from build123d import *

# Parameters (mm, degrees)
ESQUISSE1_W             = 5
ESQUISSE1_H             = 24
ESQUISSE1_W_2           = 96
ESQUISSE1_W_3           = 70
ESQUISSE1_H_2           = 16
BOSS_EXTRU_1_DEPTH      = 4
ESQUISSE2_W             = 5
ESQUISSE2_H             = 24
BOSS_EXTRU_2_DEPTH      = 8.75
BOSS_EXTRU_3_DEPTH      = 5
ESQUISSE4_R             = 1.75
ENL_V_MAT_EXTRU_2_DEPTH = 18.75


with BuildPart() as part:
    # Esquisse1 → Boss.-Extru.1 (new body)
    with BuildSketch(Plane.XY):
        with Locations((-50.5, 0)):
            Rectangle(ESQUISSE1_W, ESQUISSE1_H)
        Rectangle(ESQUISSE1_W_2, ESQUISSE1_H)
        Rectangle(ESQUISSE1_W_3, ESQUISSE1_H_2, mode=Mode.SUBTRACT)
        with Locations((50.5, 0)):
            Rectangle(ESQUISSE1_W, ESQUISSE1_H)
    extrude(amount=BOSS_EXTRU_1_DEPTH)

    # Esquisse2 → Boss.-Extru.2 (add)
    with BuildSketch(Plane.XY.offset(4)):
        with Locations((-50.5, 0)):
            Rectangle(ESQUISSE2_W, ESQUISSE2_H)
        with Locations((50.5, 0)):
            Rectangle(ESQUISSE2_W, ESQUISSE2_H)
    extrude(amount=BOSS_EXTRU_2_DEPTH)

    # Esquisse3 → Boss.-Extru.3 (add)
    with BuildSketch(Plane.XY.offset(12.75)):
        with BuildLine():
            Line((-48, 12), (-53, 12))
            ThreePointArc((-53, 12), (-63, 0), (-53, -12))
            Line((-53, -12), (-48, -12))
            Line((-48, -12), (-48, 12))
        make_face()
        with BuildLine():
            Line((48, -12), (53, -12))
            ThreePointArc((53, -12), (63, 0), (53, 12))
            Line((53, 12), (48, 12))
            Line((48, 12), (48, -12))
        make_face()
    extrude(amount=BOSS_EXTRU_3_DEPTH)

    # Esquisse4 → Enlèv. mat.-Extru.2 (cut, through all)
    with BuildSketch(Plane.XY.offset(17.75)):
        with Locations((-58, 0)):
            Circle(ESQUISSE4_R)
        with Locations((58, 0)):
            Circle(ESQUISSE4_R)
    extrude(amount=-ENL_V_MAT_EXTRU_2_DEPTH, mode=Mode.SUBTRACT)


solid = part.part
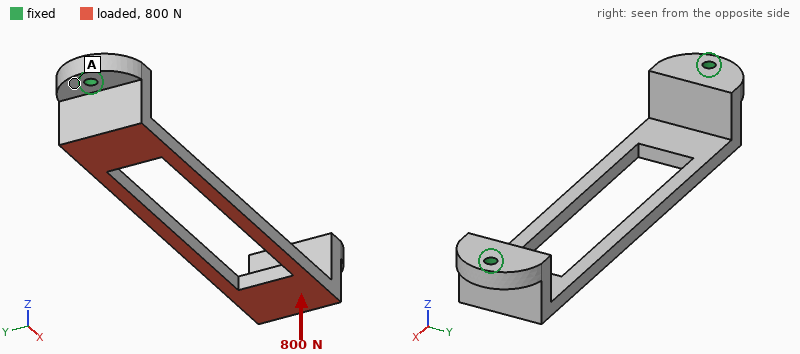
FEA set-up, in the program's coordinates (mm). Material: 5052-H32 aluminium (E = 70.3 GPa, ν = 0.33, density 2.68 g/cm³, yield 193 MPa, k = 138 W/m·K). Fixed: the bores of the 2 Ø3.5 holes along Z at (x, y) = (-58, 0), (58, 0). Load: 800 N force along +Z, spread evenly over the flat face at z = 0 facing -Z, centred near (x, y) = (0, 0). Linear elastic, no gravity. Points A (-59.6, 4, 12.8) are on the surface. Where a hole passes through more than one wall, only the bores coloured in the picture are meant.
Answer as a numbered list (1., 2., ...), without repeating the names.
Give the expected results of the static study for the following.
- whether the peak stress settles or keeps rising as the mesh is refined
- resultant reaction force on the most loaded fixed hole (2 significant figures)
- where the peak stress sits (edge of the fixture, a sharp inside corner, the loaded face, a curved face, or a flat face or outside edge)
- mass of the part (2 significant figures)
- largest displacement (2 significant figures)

1. keeps rising
2. 630 N
3. edge of the fixture
4. 29 g
5. 0.29 mm
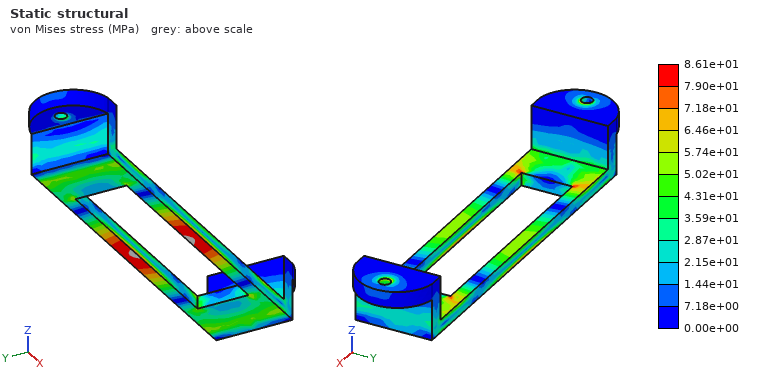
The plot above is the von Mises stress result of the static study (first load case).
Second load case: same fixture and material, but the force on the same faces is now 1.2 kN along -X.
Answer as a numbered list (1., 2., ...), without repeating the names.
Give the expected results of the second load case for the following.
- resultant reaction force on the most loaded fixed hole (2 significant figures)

1. 600 N
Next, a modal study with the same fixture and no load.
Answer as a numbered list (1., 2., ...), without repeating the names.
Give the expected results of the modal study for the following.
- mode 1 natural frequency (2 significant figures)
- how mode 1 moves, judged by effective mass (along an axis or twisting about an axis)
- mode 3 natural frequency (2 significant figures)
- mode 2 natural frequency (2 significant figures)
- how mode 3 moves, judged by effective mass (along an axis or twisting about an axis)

1. 2500 Hz
2. along Z
3. 3300 Hz
4. 2900 Hz
5. along Y
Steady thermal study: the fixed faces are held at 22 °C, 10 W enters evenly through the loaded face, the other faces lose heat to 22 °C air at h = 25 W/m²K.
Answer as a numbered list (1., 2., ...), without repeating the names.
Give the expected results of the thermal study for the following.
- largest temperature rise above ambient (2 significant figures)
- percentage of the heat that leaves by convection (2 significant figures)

1. 16 K
2. 9.9 %
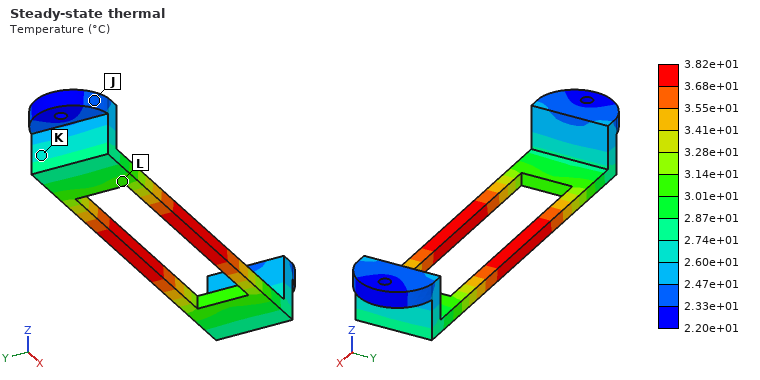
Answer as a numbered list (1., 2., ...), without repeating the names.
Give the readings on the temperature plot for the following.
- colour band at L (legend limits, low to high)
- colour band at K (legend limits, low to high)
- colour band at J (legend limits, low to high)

1. 3.01e+01 to 3.14e+01 °C
2. 2.60e+01 to 2.74e+01 °C
3. 2.33e+01 to 2.47e+01 °C
